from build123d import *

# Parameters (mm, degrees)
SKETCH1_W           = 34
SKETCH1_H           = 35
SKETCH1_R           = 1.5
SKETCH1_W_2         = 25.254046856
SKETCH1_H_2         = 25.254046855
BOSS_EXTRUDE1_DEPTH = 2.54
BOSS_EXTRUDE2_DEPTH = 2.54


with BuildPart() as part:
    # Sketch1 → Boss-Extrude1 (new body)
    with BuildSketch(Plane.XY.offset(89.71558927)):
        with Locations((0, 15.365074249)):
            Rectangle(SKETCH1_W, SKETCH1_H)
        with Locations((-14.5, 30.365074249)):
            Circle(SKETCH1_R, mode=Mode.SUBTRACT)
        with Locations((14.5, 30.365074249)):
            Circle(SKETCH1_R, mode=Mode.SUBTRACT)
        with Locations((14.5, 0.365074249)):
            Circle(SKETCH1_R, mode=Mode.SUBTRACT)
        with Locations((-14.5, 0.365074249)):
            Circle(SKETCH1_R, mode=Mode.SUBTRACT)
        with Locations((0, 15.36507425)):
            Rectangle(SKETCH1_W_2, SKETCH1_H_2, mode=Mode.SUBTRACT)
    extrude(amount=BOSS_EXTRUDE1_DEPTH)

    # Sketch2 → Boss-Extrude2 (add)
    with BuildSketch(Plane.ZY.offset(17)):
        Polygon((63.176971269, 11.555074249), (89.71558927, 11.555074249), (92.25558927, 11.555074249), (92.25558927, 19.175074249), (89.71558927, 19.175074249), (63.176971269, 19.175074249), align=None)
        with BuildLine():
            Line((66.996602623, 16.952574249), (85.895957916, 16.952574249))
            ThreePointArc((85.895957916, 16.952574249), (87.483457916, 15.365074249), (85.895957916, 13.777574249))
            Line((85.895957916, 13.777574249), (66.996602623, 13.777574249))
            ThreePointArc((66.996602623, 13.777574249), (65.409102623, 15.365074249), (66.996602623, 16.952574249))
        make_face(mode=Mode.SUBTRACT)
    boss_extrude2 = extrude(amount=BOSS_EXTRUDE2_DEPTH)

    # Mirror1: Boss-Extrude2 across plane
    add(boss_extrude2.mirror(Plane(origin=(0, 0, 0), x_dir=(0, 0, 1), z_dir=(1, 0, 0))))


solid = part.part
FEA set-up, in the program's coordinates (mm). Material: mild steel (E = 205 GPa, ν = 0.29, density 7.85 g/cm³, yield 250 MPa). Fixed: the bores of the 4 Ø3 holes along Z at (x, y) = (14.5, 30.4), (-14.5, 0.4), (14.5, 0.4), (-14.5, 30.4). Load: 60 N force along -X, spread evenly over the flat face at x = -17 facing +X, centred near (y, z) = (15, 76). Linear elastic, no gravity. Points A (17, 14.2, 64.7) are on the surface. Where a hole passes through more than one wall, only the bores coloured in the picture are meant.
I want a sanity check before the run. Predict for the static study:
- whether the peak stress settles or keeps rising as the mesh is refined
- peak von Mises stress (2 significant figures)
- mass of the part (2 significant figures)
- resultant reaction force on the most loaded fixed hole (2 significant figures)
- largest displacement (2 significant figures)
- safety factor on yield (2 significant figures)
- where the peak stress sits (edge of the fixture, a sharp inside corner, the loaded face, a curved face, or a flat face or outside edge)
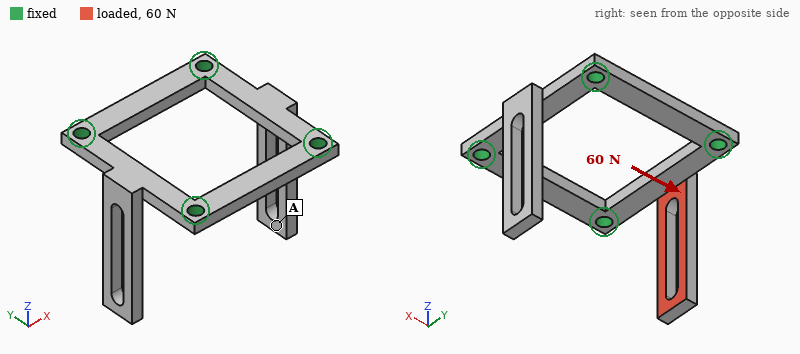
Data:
settles
170 MPa
17 g
32 N
0.25 mm
1.5
the loaded face
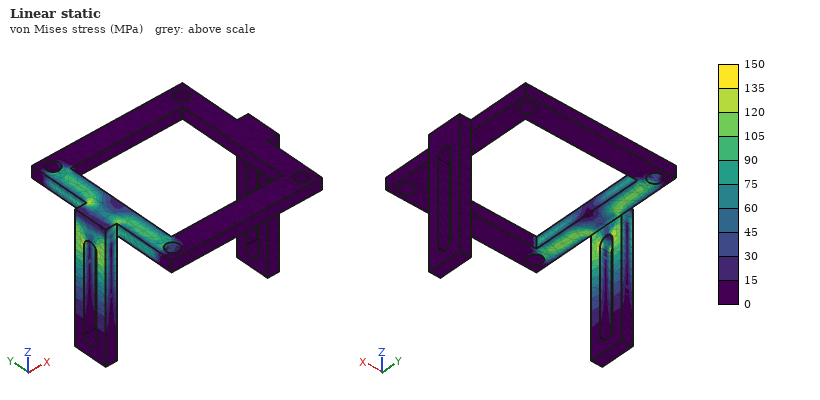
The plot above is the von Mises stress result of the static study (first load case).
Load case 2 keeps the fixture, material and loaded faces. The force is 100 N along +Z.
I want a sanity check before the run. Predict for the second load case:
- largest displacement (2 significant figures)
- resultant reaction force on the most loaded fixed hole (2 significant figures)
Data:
14 µm
51 N
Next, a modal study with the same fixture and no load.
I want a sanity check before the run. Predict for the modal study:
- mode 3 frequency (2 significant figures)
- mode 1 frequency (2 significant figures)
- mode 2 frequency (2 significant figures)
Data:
3400 Hz
1800 Hz
1800 Hz
